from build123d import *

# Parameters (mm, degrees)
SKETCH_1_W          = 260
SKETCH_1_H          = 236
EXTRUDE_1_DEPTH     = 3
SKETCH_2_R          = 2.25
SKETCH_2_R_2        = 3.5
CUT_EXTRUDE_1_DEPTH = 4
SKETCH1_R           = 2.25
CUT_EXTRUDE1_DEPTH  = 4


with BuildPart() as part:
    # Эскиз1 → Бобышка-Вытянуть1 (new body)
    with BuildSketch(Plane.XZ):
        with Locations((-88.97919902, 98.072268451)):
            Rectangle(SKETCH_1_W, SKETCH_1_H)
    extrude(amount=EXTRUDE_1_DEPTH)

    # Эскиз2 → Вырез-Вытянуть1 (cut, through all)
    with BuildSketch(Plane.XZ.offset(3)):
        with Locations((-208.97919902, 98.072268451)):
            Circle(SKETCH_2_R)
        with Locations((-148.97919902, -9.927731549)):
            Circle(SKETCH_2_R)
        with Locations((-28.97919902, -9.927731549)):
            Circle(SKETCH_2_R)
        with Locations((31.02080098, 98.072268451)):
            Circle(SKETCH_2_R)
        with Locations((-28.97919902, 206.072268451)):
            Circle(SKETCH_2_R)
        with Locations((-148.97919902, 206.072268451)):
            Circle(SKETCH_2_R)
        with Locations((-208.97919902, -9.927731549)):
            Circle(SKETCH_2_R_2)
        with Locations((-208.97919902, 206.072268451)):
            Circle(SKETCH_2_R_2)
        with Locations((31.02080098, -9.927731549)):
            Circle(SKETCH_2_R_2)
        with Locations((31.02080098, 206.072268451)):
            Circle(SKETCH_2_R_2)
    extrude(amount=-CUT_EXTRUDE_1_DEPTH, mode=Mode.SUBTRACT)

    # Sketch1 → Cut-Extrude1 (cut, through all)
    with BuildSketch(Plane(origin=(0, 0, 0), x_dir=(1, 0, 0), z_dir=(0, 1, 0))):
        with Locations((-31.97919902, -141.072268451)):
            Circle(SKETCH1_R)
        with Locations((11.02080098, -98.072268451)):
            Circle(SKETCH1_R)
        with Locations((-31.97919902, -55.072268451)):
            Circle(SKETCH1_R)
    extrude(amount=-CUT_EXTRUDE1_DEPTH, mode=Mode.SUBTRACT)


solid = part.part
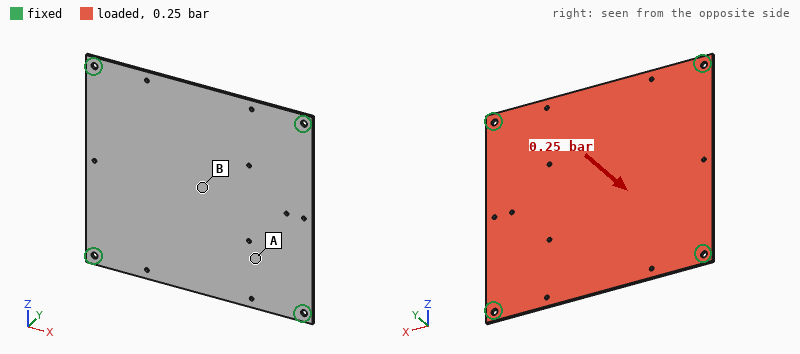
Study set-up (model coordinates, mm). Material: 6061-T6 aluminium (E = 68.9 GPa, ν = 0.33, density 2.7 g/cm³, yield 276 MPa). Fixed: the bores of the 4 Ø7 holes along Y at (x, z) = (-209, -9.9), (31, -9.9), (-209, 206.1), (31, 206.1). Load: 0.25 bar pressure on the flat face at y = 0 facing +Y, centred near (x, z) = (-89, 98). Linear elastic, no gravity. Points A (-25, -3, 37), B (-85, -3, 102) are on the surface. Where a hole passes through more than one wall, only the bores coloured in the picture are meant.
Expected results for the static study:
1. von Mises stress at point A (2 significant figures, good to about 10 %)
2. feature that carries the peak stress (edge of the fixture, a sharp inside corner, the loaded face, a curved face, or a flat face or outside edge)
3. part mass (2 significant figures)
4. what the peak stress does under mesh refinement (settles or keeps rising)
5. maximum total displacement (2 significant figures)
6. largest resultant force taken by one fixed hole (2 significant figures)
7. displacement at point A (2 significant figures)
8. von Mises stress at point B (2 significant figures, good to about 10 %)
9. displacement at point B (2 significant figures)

29 MPa
edge of the fixture
490 g
keeps rising
3.5 mm
380 N
2.1 mm
54 MPa
3.5 mm
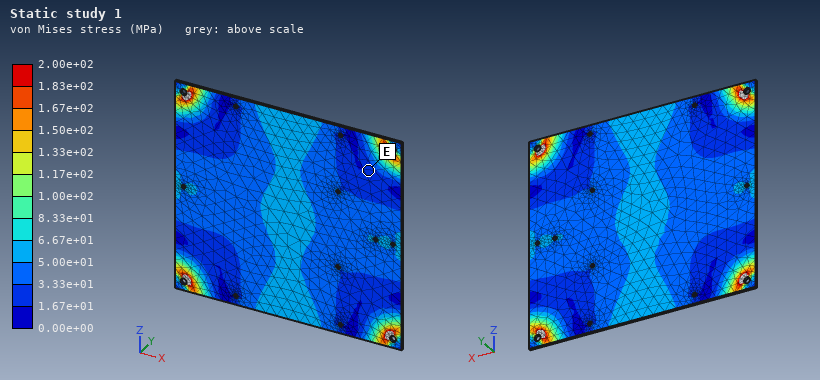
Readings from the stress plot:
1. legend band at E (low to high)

1.67e+01 to 3.33e+01 MPa
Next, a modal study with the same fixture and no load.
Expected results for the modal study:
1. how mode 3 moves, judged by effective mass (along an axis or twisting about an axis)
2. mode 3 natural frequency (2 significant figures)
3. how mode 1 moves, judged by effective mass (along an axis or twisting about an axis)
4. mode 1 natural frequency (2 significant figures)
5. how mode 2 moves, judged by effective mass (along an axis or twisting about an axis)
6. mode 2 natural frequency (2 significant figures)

twisting about Z
350 Hz
along Y
180 Hz
twisting about X
310 Hz
